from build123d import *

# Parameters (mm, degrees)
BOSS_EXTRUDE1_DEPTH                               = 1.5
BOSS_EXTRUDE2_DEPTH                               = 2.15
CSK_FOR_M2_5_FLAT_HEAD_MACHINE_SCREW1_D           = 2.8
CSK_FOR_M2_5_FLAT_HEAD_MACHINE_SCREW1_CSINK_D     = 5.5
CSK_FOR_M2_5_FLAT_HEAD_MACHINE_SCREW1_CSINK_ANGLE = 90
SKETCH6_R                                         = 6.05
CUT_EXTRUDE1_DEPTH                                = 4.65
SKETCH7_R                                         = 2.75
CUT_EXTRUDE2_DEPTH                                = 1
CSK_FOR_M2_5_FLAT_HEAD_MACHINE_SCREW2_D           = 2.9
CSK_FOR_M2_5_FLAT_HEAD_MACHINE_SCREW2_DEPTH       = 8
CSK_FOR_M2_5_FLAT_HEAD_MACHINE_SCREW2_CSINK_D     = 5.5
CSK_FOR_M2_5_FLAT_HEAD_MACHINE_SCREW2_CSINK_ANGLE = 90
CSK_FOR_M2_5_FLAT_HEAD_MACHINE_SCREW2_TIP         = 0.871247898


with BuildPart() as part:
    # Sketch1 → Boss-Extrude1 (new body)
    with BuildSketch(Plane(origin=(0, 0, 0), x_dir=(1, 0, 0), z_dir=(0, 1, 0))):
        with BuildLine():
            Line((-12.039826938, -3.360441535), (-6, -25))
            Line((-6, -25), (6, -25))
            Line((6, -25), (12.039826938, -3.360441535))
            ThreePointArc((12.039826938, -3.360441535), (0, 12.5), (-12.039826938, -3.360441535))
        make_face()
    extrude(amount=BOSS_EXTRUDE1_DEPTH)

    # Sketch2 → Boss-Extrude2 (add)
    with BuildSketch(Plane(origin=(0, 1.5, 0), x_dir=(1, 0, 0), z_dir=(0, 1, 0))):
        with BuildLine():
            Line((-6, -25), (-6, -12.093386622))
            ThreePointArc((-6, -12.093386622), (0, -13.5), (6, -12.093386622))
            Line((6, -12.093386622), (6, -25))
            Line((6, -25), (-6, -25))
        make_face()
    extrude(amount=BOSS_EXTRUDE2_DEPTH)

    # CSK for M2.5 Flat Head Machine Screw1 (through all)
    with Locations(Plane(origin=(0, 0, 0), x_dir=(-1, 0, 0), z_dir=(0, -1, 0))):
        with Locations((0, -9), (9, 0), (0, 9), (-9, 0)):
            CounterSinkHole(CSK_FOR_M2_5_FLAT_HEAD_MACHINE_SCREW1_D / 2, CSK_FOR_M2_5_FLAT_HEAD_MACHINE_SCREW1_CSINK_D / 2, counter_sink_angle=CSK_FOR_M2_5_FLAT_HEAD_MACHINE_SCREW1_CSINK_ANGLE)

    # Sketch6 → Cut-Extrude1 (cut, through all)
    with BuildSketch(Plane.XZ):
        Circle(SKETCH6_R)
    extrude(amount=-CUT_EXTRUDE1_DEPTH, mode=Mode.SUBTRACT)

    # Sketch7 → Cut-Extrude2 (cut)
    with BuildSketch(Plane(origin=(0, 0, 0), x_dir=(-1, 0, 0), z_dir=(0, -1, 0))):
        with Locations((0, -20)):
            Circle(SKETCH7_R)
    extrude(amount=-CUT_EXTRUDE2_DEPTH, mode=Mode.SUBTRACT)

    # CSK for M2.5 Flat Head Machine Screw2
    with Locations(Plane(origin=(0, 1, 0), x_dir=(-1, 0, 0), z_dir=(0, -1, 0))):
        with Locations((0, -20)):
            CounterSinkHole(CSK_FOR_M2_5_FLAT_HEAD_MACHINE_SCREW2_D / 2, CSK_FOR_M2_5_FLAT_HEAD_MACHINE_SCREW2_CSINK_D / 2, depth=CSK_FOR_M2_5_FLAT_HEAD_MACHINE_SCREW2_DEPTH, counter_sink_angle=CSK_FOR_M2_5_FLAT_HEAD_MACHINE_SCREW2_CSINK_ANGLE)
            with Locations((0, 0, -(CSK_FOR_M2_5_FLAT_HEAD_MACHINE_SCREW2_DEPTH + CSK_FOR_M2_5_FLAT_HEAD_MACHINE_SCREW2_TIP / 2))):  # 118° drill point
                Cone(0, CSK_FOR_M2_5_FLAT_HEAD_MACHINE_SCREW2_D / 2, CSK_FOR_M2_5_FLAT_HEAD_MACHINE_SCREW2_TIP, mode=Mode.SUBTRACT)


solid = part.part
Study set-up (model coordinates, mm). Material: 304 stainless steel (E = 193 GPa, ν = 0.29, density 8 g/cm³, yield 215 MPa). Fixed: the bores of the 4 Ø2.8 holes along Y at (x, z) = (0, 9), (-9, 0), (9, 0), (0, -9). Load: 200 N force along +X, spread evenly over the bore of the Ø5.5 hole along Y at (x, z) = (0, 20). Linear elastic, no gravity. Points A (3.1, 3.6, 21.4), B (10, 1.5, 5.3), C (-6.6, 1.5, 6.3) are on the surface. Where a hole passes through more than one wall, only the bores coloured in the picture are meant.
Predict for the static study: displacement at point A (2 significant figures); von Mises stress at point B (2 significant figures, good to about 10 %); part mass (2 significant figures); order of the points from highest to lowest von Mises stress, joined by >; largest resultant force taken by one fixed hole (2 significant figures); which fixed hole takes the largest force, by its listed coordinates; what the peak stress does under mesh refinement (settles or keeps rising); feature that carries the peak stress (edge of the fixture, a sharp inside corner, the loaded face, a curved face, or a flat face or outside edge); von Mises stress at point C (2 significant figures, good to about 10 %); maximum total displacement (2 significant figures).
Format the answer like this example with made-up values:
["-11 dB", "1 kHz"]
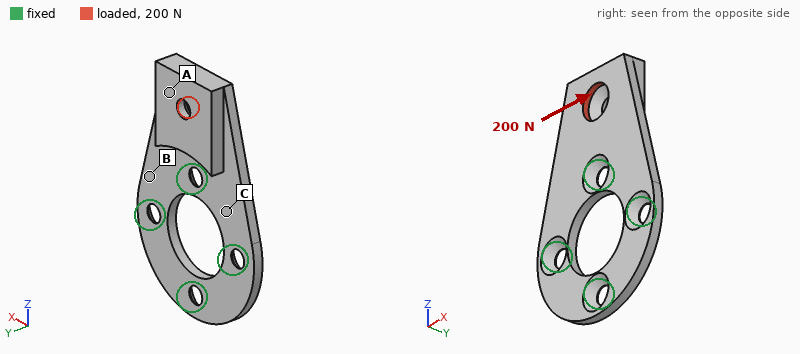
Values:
["2.9 µm", "27 MPa", "8.7 g", "B > C > A", "170 N", "(0, 9)", "keeps rising", "edge of the fixture", "15 MPa", "6.8 µm"]
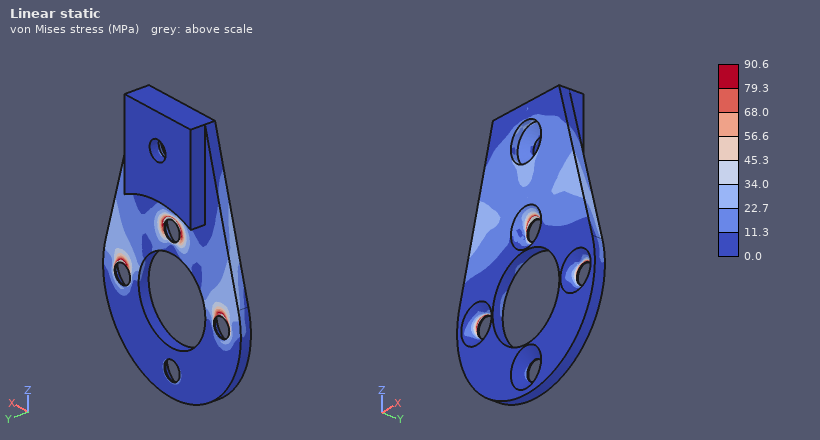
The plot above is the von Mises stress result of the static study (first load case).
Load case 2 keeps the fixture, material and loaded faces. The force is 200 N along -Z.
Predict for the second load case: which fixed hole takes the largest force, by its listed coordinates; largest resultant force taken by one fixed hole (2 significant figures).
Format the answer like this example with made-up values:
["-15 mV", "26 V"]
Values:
["(0, 9)", "77 N"]
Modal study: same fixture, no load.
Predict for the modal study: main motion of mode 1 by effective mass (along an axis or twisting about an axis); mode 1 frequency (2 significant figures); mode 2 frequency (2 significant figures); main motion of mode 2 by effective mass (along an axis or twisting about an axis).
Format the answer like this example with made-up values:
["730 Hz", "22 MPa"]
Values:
["along Y", "3200 Hz", "7300 Hz", "twisting about Z"]
